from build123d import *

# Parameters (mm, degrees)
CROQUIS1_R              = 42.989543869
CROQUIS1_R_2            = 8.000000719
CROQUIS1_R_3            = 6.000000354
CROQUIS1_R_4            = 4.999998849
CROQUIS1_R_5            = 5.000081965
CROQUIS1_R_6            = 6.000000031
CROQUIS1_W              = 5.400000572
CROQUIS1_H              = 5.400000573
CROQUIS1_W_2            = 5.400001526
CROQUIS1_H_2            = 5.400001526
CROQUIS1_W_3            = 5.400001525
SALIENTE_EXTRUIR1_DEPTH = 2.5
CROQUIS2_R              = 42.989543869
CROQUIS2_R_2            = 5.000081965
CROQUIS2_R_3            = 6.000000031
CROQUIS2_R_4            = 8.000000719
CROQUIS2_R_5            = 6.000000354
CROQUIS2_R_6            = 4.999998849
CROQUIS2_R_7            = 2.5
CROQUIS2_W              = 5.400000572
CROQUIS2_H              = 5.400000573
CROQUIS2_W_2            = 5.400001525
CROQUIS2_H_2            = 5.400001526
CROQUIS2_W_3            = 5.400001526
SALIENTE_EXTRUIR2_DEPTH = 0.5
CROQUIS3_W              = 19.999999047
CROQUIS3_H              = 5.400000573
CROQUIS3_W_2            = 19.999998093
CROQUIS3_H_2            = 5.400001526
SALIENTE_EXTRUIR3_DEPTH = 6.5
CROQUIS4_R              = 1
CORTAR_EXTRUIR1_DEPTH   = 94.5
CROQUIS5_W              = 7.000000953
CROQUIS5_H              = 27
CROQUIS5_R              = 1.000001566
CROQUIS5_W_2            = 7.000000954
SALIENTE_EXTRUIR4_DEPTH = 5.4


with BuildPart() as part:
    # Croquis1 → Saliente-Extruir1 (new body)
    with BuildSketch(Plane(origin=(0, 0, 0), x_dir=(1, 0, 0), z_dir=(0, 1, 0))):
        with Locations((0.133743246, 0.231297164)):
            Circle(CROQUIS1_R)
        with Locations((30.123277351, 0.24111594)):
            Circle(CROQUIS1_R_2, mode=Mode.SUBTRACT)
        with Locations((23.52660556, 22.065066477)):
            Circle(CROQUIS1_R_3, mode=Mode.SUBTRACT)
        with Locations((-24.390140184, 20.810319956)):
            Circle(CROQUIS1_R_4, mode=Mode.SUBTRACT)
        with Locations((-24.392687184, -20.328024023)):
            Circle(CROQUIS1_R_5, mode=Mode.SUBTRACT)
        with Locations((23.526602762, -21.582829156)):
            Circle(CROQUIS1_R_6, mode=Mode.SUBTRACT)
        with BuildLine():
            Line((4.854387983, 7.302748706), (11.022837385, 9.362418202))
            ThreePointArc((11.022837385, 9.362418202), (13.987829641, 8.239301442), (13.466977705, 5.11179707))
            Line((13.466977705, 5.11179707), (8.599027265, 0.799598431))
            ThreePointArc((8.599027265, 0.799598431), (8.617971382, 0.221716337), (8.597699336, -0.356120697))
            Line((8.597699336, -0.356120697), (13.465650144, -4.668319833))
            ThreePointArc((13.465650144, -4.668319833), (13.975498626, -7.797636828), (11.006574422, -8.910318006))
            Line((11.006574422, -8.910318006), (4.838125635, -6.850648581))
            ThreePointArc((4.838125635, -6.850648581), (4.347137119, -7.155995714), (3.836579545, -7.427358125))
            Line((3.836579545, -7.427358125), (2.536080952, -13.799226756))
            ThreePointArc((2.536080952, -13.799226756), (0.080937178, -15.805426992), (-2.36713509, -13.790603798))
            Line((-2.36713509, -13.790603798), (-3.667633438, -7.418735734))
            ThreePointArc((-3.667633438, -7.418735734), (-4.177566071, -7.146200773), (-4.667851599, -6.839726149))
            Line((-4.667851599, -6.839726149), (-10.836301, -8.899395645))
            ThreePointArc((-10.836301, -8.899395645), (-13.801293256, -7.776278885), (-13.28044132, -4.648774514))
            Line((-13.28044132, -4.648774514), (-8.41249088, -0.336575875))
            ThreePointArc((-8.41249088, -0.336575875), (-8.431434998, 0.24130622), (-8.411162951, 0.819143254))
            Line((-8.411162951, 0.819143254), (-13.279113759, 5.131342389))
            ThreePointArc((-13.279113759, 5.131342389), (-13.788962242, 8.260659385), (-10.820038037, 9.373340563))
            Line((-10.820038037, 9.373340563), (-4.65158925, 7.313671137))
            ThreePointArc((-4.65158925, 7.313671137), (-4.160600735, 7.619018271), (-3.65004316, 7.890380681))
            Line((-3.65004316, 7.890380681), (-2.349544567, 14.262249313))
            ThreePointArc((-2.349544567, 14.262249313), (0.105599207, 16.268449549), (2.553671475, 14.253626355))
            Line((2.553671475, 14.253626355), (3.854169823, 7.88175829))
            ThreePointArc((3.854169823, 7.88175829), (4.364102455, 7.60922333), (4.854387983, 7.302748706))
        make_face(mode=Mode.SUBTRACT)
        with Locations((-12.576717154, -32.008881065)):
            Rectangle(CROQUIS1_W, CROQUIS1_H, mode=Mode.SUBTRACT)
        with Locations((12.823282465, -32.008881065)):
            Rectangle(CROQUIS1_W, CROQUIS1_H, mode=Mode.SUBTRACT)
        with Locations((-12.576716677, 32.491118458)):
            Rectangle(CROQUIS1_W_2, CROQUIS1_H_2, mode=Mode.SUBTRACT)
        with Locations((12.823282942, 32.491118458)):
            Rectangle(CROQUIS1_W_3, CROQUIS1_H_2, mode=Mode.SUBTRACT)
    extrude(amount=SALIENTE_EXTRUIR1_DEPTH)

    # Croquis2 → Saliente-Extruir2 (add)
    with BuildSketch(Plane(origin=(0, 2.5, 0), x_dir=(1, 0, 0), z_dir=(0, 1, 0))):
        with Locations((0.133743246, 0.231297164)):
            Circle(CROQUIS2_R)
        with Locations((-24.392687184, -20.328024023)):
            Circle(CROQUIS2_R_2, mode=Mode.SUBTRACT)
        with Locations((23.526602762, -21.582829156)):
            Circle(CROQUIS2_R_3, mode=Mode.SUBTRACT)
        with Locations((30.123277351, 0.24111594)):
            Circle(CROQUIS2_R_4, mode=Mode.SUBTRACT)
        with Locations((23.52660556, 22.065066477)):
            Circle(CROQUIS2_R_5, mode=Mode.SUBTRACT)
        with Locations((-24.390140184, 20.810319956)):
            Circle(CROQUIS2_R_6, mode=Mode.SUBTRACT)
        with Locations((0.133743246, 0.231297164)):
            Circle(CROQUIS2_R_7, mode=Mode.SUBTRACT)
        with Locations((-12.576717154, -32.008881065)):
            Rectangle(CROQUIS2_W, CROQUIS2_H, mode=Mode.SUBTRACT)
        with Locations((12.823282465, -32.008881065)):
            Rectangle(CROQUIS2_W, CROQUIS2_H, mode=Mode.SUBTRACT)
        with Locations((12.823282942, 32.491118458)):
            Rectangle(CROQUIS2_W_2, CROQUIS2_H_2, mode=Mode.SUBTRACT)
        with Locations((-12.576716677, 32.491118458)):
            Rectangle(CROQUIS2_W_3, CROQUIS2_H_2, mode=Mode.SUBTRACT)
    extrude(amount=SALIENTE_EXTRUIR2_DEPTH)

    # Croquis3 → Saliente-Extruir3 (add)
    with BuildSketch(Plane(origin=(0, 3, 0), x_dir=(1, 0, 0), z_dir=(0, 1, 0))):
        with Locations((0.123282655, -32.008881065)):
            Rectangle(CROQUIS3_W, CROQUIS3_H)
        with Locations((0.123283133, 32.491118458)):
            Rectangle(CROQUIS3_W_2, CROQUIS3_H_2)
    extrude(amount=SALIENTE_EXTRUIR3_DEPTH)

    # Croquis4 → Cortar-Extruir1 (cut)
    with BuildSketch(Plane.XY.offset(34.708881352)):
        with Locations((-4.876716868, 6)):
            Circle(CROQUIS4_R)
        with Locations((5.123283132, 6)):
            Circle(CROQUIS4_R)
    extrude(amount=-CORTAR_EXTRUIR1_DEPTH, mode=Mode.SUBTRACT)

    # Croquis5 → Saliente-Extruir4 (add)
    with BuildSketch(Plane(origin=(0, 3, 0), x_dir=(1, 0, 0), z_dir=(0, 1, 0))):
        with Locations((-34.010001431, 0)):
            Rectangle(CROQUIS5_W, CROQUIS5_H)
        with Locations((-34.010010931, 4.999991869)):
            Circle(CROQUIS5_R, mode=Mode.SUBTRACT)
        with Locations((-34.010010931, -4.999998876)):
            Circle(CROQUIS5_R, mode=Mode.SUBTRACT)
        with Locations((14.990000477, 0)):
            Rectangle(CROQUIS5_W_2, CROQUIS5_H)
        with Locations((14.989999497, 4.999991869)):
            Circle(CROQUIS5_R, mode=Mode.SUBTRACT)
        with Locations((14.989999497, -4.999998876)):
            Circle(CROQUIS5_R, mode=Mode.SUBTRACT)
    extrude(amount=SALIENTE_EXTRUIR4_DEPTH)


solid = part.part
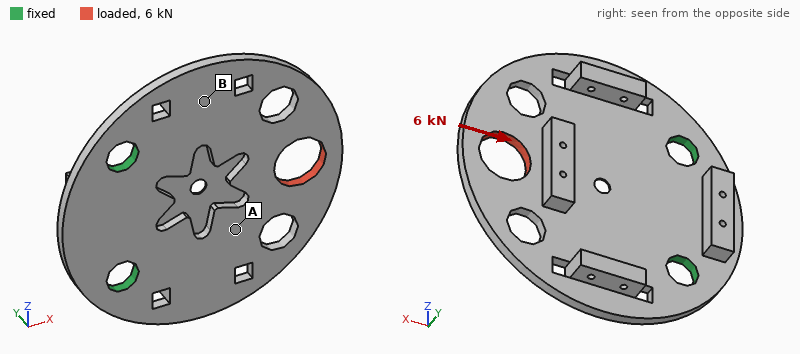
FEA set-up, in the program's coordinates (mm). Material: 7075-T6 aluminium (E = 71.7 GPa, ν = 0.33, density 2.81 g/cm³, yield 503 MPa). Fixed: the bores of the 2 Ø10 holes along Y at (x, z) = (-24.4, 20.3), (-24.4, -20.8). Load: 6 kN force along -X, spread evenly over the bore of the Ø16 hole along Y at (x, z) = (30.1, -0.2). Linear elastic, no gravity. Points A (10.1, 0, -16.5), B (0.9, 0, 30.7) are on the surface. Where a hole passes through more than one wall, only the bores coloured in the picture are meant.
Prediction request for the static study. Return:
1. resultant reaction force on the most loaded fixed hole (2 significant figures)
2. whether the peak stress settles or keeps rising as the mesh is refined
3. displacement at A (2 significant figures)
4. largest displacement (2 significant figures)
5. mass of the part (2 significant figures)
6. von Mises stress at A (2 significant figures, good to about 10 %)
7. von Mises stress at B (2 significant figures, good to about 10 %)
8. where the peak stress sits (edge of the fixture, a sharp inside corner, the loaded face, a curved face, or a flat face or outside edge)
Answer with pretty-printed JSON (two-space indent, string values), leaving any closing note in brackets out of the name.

{
  "resultant reaction force on the most loaded fixed hole": "3.0 kN",
  "whether the peak stress settles or keeps rising as the mesh is refined": "keeps rising",
  "displacement at A": "0.054 mm",
  "largest displacement": "0.24 mm",
  "mass of the part": "49 g",
  "von Mises stress at A": "81 MPa",
  "von Mises stress at B": "16 MPa",
  "where the peak stress sits": "a sharp inside corner"
}
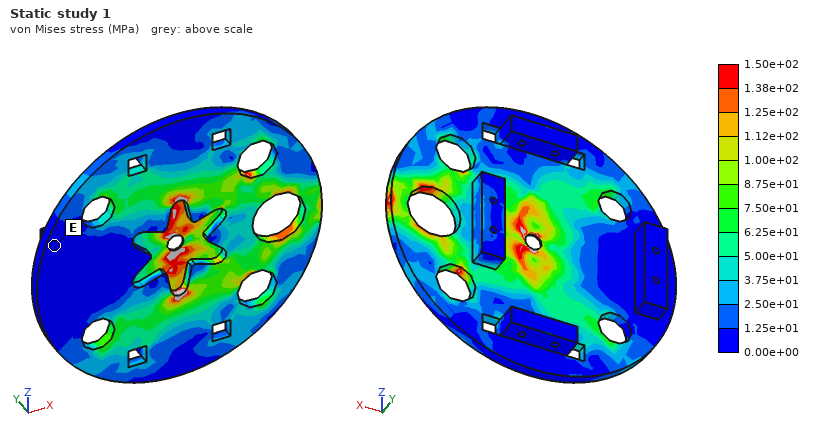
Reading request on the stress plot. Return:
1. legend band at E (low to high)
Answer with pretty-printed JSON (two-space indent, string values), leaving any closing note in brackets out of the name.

{
  "legend band at E": "0.00e+00 to 1.25e+01 MPa"
}
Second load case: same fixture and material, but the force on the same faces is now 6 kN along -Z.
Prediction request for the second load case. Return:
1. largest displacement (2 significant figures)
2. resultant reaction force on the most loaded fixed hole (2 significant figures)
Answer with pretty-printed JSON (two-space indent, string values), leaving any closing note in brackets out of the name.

{
  "largest displacement": "0.29 mm",
  "resultant reaction force on the most loaded fixed hole": "6.7 kN"
}
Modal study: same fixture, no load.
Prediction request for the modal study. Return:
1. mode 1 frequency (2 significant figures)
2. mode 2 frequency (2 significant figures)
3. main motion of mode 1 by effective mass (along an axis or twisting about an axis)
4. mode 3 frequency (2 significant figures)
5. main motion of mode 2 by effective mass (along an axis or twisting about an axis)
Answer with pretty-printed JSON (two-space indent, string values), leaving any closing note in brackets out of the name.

{
  "mode 1 frequency": "730 Hz",
  "mode 2 frequency": "1500 Hz",
  "main motion of mode 1 by effective mass": "along Y",
  "mode 3 frequency": "3000 Hz",
  "main motion of mode 2 by effective mass": "twisting about X"
}
